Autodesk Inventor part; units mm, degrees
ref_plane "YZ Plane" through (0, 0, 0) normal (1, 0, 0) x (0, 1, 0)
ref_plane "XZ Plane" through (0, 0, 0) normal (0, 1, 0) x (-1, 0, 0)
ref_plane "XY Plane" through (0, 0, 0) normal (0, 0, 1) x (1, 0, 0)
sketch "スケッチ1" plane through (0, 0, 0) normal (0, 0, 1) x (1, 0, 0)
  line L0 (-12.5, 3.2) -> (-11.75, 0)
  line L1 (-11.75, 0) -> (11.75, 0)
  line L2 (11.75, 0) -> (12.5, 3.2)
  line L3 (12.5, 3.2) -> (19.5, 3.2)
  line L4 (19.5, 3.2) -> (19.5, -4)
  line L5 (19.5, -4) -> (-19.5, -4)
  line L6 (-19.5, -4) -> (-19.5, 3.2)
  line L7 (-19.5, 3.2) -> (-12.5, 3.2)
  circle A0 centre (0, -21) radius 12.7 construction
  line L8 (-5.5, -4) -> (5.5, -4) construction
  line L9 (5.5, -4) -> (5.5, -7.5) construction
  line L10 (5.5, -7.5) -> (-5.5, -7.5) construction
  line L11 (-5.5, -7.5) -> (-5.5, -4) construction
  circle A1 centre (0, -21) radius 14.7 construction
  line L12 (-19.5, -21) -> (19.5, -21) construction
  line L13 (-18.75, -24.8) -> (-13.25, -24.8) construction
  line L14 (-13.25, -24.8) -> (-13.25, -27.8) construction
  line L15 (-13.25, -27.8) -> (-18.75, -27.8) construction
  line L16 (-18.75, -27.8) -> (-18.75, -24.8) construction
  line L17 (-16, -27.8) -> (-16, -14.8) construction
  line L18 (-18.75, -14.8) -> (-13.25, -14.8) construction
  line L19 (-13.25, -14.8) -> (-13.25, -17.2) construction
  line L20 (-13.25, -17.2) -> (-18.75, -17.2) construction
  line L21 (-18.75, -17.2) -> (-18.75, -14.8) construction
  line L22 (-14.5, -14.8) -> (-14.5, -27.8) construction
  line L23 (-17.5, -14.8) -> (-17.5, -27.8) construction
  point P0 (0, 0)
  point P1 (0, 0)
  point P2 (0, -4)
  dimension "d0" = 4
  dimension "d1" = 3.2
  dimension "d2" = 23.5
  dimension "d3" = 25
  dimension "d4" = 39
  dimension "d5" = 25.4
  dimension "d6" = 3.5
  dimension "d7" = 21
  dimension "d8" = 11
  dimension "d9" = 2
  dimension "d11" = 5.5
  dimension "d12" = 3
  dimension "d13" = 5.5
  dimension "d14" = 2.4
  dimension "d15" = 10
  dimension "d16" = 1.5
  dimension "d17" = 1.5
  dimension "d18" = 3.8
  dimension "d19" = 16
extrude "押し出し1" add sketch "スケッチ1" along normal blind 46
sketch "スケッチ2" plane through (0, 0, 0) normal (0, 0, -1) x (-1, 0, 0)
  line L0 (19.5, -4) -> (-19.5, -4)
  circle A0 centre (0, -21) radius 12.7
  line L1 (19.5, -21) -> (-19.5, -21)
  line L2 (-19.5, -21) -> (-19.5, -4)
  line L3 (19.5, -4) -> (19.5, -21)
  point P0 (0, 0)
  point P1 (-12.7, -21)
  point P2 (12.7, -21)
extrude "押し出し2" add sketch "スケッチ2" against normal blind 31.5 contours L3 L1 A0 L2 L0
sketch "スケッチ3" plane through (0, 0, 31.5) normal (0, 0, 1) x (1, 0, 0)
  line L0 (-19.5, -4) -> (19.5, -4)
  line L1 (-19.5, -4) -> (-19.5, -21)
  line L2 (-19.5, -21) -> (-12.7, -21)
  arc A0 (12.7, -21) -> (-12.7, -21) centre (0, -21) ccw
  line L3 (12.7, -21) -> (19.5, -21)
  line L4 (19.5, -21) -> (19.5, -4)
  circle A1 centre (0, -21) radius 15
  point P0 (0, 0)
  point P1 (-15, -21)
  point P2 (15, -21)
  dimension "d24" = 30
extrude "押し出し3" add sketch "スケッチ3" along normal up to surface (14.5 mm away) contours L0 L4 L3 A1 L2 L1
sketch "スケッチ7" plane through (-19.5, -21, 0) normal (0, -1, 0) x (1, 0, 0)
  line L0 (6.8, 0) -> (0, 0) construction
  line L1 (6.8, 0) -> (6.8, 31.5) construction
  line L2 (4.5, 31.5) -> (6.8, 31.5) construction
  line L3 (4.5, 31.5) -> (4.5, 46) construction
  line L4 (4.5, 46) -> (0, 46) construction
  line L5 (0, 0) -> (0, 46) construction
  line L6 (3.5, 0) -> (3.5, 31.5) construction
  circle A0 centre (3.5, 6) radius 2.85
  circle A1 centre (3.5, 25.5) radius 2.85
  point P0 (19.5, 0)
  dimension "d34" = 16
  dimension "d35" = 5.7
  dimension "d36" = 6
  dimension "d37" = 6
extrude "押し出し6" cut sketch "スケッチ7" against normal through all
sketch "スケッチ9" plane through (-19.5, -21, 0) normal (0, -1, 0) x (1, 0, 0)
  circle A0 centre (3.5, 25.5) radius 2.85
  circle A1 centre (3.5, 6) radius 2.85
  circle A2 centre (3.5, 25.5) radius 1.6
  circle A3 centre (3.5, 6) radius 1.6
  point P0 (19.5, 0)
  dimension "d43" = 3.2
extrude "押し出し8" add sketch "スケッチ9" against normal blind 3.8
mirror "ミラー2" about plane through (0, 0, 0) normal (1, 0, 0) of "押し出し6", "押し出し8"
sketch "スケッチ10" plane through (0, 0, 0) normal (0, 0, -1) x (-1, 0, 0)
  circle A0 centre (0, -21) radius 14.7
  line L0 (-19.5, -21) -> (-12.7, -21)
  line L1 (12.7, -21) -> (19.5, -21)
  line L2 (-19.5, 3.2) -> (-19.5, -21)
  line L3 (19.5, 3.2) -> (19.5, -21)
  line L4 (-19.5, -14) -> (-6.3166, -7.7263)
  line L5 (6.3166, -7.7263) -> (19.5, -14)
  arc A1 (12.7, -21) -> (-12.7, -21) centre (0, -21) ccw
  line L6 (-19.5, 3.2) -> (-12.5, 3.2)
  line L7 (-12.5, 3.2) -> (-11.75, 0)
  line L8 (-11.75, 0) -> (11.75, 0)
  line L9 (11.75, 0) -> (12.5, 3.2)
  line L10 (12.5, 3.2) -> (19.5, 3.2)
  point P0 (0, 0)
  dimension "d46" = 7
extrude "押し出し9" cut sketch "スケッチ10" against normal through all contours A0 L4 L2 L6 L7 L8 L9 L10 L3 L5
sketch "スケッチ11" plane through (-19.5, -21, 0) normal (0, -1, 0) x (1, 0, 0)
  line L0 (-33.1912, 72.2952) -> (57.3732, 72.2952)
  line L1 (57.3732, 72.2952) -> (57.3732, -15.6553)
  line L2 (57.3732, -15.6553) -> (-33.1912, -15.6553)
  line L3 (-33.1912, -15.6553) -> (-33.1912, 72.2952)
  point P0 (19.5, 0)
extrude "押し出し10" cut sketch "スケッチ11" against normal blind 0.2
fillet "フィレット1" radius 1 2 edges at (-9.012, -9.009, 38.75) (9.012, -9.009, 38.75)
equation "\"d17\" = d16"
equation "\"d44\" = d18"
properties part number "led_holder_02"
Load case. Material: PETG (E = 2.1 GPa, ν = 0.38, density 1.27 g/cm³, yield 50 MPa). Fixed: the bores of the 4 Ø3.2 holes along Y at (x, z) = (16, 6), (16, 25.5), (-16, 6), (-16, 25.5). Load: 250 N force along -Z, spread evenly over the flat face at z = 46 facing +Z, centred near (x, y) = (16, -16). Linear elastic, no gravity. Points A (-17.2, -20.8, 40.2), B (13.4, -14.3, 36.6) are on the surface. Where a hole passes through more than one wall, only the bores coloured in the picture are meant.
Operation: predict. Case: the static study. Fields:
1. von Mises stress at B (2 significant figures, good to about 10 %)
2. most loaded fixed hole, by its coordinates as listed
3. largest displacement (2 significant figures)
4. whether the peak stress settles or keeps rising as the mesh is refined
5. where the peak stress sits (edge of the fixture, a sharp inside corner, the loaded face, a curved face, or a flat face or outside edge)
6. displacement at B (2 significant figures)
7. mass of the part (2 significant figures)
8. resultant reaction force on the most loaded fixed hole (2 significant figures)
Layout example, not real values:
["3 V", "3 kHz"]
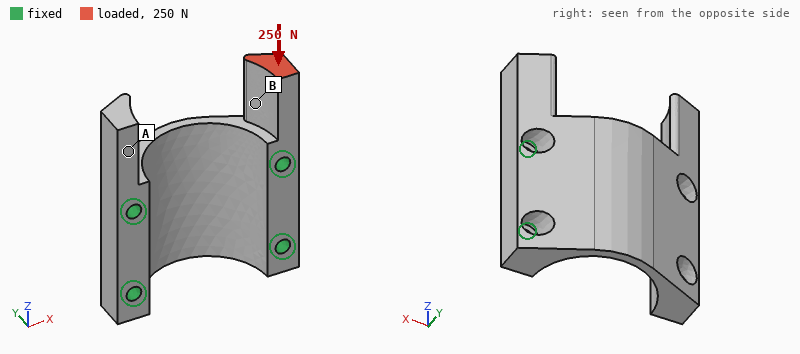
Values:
["5.6 MPa", "(16, 25.5)", "0.21 mm", "keeps rising", "edge of the fixture", "0.10 mm", "8.5 g", "200 N"]
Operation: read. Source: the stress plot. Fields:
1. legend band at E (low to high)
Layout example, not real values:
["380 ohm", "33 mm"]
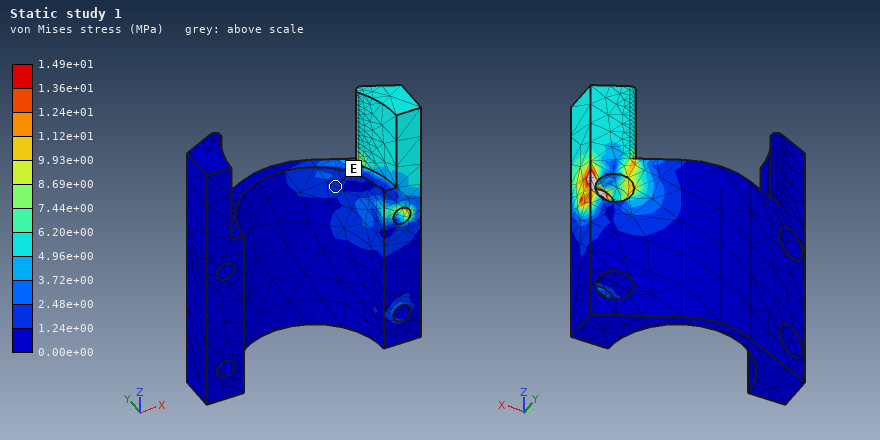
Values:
["1.24e+00 to 2.48e+00 MPa"]
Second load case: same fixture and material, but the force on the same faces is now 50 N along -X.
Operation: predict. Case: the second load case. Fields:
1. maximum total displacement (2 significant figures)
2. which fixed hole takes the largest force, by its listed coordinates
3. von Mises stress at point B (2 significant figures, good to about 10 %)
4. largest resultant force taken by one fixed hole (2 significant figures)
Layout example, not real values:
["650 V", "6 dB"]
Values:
["0.62 mm", "(16, 25.5)", "11 MPa", "64 N"]
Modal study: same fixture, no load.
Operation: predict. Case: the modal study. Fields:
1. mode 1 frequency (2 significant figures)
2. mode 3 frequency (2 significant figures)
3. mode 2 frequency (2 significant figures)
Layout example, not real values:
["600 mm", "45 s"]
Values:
["2500 Hz", "3700 Hz", "2500 Hz"]
